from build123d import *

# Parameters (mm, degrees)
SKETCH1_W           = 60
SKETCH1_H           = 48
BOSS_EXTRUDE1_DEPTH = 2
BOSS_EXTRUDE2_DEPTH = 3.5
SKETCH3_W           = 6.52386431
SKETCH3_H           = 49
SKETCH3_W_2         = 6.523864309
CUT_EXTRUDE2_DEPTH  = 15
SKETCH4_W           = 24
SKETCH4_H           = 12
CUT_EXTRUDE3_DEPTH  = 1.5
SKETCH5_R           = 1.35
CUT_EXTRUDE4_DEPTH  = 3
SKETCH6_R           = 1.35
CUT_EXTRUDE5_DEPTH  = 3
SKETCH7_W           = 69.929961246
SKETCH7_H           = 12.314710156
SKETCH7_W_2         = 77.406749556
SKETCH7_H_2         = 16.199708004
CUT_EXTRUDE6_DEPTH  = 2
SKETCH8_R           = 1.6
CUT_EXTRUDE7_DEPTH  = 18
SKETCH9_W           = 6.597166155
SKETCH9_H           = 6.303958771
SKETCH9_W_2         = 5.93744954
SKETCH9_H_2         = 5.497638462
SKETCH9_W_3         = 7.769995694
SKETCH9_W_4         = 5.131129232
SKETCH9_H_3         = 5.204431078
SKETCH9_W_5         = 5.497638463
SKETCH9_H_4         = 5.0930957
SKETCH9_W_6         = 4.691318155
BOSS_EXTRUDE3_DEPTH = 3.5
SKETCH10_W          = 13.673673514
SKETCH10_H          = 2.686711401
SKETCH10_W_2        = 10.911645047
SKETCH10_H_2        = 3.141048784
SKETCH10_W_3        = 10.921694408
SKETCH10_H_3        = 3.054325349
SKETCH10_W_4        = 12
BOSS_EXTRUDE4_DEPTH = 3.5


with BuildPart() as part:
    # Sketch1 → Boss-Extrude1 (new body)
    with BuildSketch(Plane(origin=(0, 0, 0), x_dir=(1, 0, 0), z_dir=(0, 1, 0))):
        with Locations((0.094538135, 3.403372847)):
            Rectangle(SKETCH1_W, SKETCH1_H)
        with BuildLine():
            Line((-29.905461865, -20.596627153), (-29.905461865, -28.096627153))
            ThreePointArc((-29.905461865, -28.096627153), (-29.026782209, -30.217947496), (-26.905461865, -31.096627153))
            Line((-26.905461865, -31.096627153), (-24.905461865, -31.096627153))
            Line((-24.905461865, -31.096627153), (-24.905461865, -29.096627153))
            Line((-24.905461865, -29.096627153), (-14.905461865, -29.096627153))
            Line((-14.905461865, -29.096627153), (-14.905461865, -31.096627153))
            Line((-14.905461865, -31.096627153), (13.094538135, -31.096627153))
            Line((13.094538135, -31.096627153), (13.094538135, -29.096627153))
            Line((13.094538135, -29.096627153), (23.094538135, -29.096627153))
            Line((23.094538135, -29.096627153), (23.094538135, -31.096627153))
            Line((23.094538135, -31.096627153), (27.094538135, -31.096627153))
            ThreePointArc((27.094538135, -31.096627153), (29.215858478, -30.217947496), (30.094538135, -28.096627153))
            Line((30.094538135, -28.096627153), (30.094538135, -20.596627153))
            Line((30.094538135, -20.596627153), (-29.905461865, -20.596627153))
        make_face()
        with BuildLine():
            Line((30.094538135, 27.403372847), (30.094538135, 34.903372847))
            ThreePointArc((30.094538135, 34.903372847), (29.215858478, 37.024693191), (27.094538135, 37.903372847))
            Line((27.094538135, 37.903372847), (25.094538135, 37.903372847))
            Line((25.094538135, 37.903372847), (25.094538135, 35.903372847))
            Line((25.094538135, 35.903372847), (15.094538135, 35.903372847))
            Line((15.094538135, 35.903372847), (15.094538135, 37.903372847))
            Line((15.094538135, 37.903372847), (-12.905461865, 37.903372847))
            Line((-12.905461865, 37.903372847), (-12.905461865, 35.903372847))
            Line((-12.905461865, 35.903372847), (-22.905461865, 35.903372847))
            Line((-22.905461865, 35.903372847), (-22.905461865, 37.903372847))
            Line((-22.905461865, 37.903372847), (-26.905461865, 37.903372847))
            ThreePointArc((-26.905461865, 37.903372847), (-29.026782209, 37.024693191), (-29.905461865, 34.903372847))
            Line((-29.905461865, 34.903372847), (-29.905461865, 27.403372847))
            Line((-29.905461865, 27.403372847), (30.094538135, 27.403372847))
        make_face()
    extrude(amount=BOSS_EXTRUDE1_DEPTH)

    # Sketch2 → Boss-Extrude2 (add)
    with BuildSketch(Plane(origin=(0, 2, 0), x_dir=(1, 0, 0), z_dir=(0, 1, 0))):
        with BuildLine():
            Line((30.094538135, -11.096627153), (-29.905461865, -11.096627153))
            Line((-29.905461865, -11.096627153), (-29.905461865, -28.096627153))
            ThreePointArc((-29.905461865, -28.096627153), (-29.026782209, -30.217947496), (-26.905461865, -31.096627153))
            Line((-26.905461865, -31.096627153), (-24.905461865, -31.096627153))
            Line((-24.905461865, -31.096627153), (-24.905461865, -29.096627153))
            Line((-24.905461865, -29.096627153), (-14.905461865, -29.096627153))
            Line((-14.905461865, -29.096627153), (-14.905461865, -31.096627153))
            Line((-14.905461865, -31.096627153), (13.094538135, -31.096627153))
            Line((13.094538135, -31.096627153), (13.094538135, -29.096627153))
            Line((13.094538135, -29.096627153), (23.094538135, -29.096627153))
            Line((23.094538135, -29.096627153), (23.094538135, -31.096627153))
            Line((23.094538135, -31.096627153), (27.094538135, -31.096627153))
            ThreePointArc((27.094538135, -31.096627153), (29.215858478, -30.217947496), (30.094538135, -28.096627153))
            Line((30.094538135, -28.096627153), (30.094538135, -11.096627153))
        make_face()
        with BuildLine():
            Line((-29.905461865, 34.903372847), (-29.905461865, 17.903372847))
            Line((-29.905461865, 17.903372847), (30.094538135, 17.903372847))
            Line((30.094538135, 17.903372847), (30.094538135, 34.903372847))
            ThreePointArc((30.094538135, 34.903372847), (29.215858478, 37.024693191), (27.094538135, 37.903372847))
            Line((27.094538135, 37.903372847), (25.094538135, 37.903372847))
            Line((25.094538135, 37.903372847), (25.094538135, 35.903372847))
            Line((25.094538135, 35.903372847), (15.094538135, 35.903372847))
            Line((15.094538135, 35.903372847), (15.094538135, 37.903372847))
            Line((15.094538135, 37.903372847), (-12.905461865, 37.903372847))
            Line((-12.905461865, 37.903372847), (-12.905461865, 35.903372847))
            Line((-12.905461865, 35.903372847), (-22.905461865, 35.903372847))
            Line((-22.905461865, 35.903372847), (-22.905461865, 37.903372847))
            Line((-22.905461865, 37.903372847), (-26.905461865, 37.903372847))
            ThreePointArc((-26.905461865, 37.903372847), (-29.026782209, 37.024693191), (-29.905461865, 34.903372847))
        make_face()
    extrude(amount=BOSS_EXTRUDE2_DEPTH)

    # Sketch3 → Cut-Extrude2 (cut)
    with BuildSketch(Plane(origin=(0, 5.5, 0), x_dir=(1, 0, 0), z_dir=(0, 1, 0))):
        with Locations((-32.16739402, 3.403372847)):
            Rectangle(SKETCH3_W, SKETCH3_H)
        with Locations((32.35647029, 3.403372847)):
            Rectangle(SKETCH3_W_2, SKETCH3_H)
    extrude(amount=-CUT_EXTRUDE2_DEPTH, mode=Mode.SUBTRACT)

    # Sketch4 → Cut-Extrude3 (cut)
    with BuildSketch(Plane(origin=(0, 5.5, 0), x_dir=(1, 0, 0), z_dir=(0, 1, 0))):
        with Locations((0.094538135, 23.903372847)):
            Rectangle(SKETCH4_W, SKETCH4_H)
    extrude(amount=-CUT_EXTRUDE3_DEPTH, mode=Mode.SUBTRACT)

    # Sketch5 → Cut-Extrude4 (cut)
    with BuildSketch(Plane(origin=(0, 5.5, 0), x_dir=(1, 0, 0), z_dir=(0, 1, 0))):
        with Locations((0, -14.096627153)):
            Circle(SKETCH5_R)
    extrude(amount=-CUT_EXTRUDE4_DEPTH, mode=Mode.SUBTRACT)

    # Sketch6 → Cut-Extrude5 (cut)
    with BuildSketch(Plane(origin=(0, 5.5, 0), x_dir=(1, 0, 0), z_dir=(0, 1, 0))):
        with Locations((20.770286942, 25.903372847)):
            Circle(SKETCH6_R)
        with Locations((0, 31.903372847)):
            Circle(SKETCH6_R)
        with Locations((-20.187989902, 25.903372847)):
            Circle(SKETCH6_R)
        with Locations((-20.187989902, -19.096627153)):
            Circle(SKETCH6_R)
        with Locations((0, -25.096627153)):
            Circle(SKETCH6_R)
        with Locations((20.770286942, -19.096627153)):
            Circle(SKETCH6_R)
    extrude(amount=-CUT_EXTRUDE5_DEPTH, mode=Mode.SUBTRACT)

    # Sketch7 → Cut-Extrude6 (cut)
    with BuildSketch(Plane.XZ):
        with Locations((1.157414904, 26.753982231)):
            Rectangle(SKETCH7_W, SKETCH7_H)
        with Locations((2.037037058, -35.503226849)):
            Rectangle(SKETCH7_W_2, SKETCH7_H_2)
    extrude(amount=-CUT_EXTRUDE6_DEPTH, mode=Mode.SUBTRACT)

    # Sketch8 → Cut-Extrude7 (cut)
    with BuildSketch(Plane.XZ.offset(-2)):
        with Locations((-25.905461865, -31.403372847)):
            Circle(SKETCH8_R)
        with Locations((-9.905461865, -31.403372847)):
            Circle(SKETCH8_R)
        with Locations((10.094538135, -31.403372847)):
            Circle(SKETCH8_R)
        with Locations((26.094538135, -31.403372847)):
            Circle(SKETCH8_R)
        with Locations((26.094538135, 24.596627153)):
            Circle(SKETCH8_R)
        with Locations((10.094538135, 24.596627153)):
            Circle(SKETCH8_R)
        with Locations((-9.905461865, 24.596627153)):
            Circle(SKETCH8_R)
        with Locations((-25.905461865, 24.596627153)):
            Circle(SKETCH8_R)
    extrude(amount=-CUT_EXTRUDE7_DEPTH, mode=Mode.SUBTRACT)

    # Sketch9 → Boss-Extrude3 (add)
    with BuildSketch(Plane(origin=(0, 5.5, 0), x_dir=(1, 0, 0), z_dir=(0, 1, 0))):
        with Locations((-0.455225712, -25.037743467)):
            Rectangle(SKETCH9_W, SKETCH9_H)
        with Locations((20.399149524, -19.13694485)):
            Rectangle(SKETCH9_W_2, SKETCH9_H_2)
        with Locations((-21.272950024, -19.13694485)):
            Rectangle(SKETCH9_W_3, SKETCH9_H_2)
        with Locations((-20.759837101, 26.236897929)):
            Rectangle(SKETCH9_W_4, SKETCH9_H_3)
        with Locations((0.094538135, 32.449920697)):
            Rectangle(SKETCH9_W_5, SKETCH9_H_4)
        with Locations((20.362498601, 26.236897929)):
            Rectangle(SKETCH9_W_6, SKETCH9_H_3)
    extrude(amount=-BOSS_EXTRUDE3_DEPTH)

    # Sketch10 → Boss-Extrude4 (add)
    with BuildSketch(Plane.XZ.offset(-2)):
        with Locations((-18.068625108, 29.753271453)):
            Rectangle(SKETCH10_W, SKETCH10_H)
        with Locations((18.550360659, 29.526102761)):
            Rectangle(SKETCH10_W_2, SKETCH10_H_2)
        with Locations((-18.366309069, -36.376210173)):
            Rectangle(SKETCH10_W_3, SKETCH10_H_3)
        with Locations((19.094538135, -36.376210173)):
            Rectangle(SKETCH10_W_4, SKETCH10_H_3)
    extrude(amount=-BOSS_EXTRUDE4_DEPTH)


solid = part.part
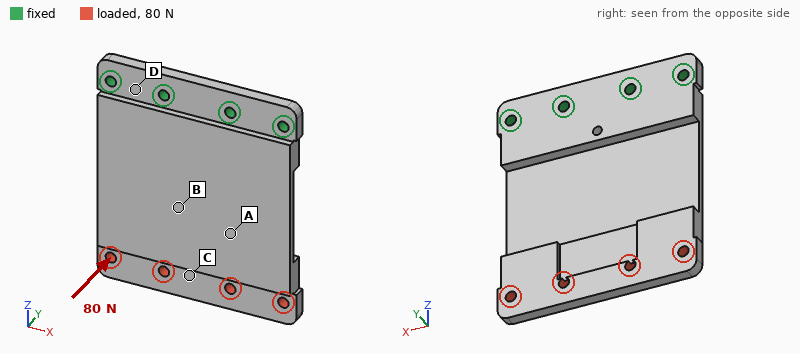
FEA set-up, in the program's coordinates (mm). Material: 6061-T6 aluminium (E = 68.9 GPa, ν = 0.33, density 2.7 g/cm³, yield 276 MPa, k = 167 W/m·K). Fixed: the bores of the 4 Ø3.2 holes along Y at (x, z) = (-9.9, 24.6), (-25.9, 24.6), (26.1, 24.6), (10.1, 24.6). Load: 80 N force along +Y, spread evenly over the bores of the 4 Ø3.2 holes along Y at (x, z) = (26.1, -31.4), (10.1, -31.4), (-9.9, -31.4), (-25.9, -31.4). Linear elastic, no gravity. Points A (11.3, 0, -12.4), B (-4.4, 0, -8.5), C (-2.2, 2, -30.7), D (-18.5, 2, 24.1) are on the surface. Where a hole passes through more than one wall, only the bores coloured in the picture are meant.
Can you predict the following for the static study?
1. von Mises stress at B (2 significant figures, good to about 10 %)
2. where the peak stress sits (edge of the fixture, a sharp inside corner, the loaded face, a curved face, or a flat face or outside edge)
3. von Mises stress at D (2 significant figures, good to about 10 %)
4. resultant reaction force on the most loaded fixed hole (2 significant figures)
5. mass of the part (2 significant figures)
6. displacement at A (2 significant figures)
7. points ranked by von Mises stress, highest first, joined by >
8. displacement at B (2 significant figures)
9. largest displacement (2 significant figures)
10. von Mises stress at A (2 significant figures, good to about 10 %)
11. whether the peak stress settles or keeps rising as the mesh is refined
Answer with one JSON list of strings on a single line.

["42 MPa", "edge of the fixture", "16 MPa", "49 N", "35 g", "0.36 mm", "B > A > D > C", "0.27 mm", "1.0 mm", "35 MPa", "keeps rising"]
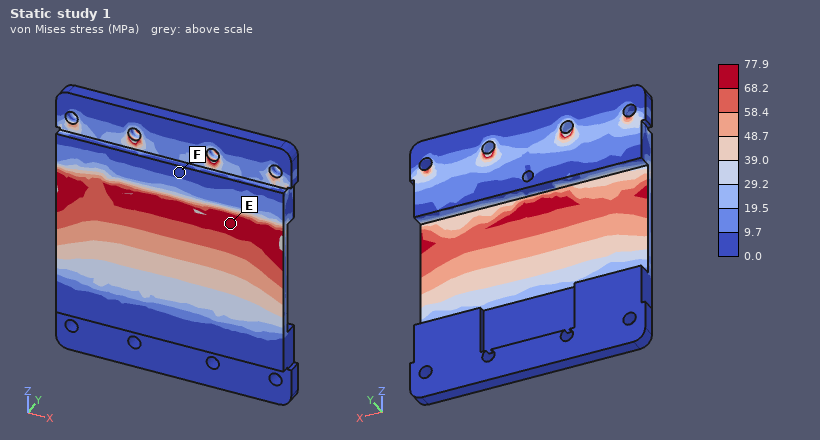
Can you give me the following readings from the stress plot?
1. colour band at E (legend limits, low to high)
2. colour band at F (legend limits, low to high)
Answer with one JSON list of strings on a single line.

["68.2 to 77.9 MPa", "0.0 to 9.7 MPa"]
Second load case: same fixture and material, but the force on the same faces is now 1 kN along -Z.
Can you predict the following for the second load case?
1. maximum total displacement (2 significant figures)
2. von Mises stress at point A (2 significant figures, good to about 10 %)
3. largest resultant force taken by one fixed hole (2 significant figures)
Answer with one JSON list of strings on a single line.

["1.0 mm", "54 MPa", "290 N"]
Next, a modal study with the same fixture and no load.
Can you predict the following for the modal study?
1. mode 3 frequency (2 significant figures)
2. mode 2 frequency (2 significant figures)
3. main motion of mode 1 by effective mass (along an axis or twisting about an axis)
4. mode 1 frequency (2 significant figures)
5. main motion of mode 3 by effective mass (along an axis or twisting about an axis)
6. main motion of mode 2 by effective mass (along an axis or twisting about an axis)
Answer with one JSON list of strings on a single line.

["3300 Hz", "1300 Hz", "along Y", "480 Hz", "along Y", "twisting about Z"]
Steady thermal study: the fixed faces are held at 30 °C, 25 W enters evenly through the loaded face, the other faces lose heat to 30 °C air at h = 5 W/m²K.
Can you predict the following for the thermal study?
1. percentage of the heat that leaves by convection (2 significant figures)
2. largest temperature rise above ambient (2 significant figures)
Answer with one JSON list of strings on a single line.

["5.2 %", "58 K"]
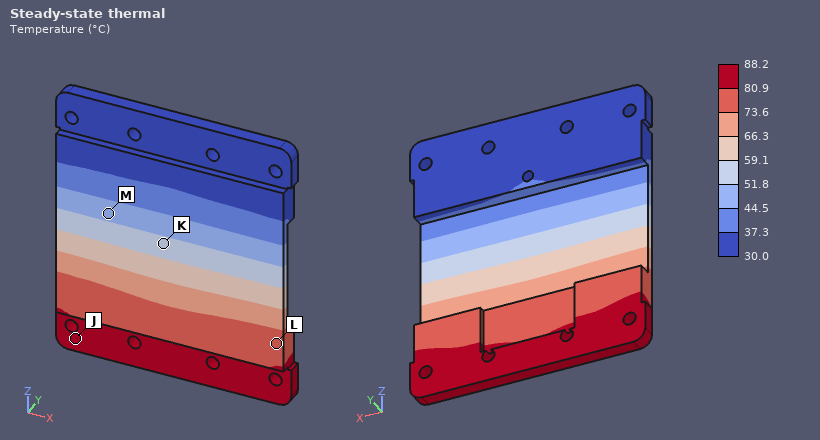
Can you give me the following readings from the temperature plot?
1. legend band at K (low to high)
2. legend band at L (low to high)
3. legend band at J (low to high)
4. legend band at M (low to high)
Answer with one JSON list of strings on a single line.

["51.8 to 59.1 °C", "73.6 to 80.9 °C", "80.9 to 88.2 °C", "44.5 to 51.8 °C"]
